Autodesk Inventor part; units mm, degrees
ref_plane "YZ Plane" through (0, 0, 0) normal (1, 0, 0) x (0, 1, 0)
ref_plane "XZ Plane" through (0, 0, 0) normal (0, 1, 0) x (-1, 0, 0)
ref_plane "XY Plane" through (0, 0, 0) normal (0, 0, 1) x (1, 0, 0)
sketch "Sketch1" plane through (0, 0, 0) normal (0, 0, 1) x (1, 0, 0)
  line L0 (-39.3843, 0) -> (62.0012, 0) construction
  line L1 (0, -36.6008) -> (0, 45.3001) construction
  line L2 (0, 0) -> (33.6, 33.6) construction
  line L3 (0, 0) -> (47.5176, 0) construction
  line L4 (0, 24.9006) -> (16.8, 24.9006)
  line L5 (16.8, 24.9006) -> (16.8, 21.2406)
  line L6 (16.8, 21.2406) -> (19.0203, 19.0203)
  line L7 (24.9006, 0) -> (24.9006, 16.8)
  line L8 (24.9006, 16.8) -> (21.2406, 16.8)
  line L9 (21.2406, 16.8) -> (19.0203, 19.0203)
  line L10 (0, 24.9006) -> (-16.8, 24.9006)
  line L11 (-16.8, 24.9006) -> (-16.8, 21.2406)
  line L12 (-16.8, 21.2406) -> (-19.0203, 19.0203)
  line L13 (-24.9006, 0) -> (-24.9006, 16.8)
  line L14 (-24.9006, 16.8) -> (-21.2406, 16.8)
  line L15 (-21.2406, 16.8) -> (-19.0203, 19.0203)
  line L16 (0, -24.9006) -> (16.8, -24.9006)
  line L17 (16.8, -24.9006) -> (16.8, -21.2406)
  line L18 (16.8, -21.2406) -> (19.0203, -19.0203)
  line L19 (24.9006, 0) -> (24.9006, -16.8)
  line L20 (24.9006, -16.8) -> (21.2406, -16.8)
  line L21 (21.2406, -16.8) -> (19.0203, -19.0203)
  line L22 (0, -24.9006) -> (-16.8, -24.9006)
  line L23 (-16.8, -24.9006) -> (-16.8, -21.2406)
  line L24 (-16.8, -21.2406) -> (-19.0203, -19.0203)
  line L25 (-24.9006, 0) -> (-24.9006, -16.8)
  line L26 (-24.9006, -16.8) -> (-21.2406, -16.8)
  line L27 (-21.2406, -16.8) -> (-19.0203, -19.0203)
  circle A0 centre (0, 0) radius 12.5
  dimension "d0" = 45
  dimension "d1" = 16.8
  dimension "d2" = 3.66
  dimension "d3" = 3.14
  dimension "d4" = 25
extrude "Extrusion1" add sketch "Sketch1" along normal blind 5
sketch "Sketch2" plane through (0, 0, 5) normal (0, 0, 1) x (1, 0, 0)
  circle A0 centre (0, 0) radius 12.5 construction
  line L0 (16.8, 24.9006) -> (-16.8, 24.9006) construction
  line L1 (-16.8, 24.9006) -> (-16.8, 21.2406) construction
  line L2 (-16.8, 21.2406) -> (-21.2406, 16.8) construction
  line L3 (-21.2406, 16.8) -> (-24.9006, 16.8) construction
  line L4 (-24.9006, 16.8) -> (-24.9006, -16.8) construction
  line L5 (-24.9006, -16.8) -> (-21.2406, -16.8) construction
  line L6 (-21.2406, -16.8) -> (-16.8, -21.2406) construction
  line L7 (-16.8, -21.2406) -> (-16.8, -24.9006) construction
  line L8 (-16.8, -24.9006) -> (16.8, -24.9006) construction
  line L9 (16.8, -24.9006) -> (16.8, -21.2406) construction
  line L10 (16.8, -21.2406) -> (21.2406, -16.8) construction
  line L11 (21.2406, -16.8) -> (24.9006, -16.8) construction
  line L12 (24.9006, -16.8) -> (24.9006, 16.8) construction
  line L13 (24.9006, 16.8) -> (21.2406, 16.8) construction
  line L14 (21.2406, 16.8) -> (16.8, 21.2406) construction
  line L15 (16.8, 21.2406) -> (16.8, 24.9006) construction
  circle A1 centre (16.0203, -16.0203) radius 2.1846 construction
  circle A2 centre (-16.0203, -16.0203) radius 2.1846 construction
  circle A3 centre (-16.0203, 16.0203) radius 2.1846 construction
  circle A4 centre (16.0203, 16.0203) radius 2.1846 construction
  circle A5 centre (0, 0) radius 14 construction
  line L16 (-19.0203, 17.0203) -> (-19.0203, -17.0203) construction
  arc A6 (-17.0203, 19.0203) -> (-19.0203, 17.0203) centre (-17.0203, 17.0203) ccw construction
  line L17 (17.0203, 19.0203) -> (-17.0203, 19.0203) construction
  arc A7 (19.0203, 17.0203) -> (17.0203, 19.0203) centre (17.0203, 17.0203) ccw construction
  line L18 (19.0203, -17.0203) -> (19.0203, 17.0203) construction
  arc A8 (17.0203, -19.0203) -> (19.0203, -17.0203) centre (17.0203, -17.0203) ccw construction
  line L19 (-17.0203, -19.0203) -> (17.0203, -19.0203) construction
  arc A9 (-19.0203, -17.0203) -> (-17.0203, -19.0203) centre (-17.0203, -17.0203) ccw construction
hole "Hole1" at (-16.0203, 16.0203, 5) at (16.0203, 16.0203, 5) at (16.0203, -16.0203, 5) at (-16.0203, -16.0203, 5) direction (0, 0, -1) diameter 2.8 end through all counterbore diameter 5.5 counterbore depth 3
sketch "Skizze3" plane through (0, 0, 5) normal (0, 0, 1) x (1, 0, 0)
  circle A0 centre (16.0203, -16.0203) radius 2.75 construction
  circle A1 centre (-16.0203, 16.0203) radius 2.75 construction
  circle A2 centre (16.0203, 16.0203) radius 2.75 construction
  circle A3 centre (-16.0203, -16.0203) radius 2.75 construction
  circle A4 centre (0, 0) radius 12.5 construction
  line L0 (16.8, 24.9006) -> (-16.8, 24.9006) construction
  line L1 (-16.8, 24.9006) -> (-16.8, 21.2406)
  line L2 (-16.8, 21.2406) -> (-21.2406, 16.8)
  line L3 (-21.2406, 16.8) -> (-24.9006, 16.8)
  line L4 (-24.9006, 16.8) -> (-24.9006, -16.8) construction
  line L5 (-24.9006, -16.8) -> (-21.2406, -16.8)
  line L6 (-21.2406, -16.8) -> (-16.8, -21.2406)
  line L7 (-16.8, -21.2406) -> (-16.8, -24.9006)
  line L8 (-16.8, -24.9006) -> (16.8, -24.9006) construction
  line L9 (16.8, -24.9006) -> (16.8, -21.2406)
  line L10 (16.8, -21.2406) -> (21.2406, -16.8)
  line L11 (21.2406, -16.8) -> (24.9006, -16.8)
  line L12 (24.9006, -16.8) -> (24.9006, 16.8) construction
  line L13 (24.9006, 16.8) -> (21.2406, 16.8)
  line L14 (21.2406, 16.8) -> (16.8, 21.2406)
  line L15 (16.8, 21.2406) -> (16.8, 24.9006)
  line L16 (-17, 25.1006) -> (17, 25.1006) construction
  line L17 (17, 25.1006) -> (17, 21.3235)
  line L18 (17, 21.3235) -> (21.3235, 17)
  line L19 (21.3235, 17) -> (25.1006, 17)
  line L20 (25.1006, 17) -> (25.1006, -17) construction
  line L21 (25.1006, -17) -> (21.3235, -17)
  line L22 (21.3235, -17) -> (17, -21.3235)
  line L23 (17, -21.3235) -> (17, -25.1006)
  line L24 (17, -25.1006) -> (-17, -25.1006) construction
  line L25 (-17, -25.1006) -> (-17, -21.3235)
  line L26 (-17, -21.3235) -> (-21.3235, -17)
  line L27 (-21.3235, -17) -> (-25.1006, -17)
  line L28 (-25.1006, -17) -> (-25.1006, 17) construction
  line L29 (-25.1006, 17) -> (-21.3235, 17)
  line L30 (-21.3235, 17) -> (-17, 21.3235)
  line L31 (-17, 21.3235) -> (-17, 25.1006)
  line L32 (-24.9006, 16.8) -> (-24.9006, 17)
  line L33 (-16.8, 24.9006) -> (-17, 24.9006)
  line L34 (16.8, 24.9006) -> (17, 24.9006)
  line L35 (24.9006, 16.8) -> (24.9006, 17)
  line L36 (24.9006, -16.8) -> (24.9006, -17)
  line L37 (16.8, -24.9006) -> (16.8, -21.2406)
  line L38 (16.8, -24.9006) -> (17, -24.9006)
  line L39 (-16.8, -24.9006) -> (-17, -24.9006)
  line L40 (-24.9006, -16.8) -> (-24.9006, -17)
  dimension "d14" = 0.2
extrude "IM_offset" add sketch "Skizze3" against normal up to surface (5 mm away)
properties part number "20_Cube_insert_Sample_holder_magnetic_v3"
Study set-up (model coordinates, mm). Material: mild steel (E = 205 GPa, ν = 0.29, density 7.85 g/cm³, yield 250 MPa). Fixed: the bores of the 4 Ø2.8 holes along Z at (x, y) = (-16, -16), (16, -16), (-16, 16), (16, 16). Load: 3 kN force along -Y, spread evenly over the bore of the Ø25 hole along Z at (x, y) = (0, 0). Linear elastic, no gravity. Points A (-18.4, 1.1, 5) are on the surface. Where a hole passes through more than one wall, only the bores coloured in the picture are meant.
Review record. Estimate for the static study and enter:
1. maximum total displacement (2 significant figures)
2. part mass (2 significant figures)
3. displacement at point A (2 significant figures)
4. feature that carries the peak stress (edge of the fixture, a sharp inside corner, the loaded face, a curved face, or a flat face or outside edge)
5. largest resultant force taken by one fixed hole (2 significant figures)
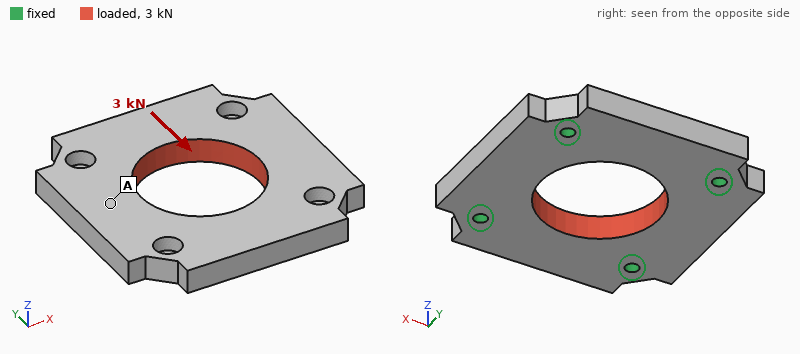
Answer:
2.7 µm
67 g
0.81 µm
edge of the fixture
750 N
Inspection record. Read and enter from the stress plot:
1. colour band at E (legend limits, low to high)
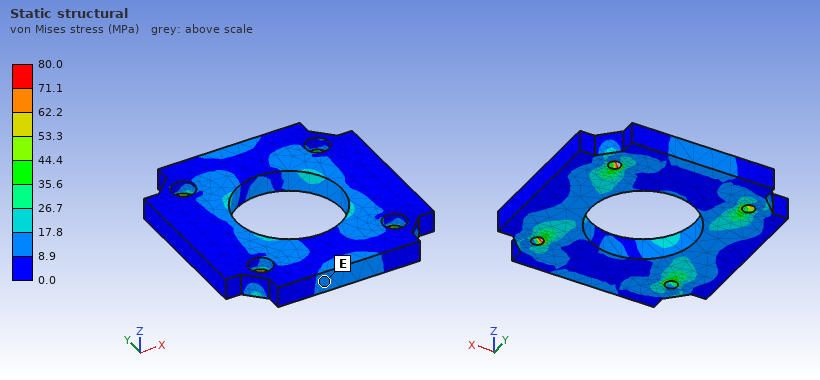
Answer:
8.9 to 17.8 MPa
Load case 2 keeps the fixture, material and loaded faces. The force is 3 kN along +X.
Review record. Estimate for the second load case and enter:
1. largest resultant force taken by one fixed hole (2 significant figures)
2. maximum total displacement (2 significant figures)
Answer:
750 N
2.7 µm
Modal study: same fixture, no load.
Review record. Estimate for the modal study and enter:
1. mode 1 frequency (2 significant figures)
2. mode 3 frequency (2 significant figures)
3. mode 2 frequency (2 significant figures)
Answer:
12 kHz
15 kHz
15 kHz
